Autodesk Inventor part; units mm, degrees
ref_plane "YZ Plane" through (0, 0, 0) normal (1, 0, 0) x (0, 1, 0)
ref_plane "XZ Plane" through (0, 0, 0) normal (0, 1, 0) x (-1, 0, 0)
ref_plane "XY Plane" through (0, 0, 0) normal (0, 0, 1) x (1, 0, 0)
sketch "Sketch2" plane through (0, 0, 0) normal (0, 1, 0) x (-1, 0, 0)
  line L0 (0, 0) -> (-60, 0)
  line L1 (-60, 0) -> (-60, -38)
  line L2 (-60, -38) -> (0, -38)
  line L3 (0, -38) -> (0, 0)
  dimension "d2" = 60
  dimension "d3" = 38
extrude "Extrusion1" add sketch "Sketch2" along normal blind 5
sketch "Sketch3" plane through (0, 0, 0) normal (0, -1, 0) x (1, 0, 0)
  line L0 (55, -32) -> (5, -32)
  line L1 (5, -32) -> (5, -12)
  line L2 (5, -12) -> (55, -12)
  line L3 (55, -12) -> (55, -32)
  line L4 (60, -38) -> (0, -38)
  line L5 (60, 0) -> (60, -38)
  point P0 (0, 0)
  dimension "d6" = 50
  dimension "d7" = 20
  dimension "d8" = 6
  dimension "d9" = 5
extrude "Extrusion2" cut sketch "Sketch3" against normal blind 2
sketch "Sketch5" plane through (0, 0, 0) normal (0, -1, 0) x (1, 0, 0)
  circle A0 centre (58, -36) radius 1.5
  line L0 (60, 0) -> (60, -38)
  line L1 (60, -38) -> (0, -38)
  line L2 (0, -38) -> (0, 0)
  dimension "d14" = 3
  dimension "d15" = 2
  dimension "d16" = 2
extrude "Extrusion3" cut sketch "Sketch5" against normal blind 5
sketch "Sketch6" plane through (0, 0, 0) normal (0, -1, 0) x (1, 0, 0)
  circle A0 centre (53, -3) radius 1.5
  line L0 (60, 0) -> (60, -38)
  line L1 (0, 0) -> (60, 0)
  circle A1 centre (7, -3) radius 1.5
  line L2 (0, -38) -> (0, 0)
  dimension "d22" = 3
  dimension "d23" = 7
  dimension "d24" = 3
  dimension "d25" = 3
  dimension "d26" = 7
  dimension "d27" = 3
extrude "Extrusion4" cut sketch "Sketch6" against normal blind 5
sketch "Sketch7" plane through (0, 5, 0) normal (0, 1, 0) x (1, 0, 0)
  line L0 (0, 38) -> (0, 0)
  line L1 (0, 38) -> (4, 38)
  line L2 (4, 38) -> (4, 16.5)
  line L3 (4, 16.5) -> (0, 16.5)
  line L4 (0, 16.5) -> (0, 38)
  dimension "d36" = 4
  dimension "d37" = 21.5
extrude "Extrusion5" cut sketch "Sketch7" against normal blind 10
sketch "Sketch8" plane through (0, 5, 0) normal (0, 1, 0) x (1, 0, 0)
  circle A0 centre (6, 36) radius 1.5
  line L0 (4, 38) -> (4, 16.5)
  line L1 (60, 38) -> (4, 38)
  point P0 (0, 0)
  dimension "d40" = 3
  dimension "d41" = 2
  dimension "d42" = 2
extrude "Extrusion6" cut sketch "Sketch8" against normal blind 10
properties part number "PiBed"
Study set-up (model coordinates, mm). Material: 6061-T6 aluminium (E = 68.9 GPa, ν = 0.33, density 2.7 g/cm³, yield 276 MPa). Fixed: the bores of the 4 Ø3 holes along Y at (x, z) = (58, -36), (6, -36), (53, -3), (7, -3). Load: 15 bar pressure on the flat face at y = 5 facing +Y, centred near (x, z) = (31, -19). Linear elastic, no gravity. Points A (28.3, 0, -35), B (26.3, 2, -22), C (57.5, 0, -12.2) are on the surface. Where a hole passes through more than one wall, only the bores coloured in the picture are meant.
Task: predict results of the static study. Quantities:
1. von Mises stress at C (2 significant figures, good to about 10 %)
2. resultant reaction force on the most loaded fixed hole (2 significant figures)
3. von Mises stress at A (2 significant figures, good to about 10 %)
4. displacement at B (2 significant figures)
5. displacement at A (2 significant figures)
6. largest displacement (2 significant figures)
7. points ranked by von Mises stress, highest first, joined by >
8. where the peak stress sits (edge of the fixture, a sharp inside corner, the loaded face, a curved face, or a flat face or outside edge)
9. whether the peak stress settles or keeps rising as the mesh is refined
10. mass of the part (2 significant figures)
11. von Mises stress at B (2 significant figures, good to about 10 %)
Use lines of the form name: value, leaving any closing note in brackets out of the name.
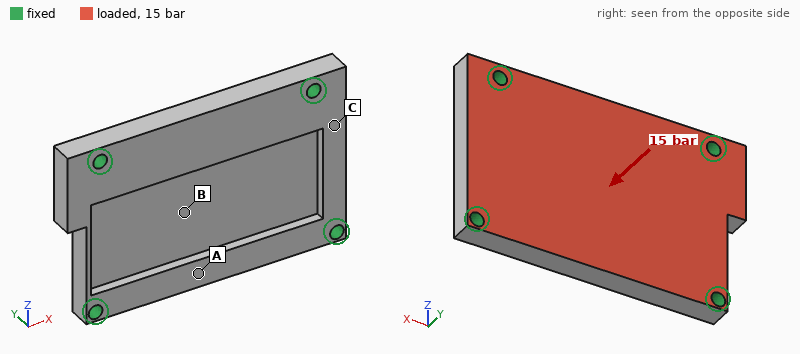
von Mises stress at C: 22 MPa
resultant reaction force on the most loaded fixed hole: 1.0 kN
von Mises stress at A: 71 MPa
displacement at B: 84 µm
displacement at A: 73 µm
largest displacement: 89 µm
points ranked by von Mises stress, highest first, joined by >: A > B > C
where the peak stress sits: edge of the fixture
whether the peak stress settles or keeps rising as the mesh is refined: keeps rising
mass of the part: 24 g
von Mises stress at B: 43 MPa
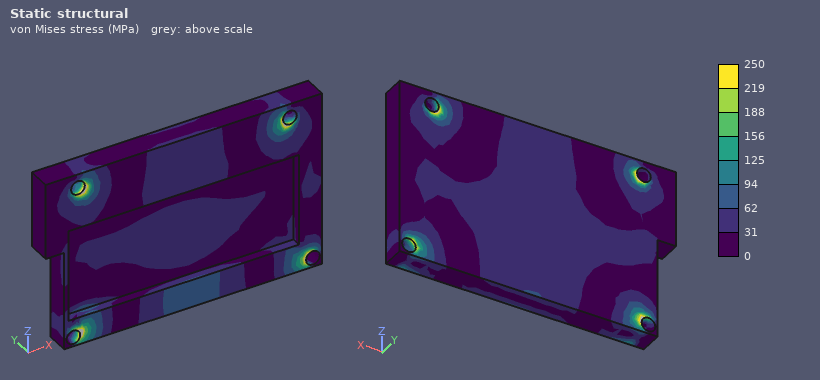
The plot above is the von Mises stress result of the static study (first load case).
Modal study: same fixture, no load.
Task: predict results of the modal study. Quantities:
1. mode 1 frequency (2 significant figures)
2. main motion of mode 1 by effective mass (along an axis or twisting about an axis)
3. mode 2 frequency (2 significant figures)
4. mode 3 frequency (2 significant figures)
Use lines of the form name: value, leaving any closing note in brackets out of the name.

mode 1 frequency: 8000 Hz
main motion of mode 1 by effective mass: along Y
mode 2 frequency: 12 kHz
mode 3 frequency: 17 kHz
